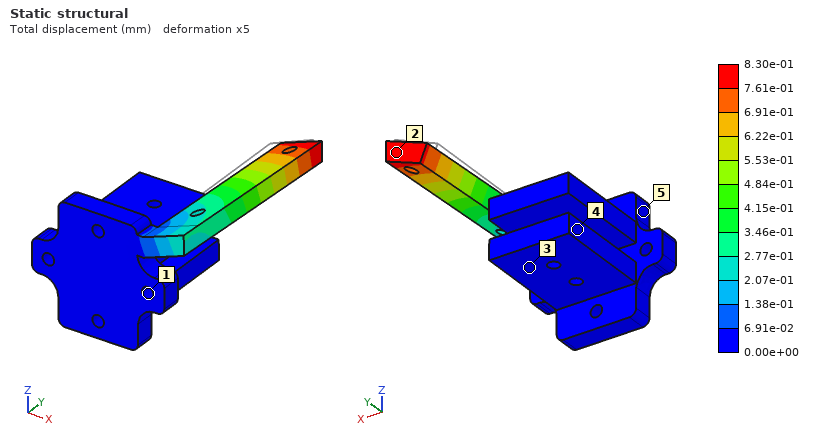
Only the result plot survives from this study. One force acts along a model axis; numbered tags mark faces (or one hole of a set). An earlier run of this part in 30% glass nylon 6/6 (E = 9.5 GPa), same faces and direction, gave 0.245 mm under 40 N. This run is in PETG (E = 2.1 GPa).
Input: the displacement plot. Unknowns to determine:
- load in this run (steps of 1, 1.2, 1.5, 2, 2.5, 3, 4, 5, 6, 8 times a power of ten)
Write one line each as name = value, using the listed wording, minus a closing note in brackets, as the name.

load in this run = 30 N
